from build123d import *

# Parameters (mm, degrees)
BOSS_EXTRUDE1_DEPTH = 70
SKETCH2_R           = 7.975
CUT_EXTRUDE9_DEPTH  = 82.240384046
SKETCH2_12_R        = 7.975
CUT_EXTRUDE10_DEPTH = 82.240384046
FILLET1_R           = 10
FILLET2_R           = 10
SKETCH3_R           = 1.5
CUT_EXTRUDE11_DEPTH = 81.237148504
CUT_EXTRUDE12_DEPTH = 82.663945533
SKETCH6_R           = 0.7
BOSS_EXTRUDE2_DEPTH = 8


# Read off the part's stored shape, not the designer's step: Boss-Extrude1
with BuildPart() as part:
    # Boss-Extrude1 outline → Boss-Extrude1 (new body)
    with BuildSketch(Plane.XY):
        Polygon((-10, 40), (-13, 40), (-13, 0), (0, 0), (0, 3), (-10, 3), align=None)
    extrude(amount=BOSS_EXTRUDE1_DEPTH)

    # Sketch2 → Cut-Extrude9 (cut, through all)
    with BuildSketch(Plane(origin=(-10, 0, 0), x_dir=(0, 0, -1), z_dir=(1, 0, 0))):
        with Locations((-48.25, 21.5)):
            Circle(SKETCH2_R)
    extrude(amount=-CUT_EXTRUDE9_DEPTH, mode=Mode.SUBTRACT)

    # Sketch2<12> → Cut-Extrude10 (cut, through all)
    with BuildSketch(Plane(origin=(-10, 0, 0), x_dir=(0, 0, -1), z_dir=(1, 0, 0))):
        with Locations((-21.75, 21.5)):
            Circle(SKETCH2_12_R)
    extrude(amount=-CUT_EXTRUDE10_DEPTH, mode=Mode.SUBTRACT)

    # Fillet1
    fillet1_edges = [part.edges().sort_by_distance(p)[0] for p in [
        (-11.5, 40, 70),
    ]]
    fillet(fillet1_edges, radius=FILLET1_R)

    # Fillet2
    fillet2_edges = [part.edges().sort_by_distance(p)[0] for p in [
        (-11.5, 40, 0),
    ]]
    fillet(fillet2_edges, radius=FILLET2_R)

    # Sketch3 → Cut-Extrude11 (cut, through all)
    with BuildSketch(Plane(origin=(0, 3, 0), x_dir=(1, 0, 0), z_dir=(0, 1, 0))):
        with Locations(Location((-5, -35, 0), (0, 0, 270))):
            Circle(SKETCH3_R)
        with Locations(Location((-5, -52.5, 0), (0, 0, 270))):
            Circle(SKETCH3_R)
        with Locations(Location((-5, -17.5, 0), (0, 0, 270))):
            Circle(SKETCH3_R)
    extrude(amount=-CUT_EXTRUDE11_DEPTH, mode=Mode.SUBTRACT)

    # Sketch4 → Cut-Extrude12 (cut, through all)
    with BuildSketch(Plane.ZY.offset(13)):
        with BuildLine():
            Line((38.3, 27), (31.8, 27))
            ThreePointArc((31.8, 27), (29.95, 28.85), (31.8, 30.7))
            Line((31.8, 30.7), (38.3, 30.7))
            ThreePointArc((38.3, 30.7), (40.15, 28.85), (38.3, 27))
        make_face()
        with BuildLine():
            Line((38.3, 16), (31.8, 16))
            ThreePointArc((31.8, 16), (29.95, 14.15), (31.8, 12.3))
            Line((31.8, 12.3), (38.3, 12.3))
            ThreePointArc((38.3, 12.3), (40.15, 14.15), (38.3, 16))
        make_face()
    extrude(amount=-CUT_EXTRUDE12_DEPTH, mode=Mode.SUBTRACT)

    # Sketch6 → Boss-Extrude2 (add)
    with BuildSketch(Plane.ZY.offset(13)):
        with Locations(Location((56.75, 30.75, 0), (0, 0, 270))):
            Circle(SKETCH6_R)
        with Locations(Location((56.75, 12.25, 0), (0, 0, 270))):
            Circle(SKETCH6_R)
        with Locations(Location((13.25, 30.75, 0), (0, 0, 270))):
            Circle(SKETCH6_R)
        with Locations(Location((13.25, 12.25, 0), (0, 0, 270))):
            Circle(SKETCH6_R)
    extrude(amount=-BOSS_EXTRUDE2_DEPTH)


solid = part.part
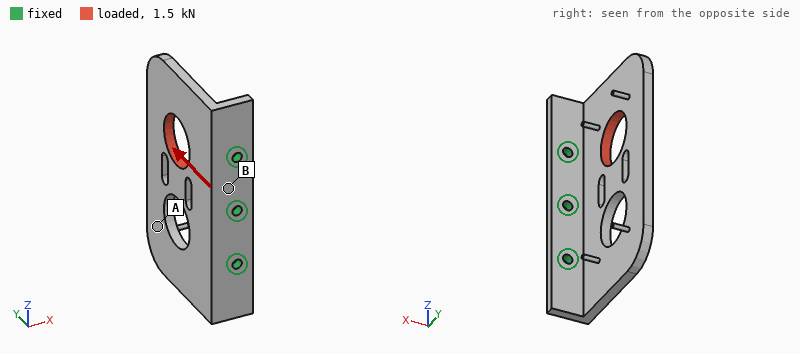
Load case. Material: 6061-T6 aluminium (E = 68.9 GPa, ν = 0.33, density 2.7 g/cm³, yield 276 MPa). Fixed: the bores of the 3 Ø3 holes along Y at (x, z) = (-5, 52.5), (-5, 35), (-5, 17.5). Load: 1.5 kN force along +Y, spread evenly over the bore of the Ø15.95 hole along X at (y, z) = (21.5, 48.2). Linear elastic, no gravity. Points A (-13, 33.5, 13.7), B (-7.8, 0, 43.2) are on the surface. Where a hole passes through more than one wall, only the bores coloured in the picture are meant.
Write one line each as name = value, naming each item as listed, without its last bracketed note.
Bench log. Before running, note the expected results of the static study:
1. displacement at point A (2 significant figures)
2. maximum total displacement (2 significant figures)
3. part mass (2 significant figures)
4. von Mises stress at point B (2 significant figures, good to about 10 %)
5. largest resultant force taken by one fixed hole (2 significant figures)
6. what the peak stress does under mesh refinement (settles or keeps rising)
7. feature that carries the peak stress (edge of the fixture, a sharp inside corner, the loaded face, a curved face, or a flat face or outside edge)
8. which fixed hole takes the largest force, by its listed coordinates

displacement at point A = 0.090 mm
maximum total displacement = 0.23 mm
part mass = 24 g
von Mises stress at point B = 44 MPa
largest resultant force taken by one fixed hole = 1.1 kN
what the peak stress does under mesh refinement = keeps rising
feature that carries the peak stress = edge of the fixture
which fixed hole takes the largest force, by its listed coordinates = (-5, 52.5)
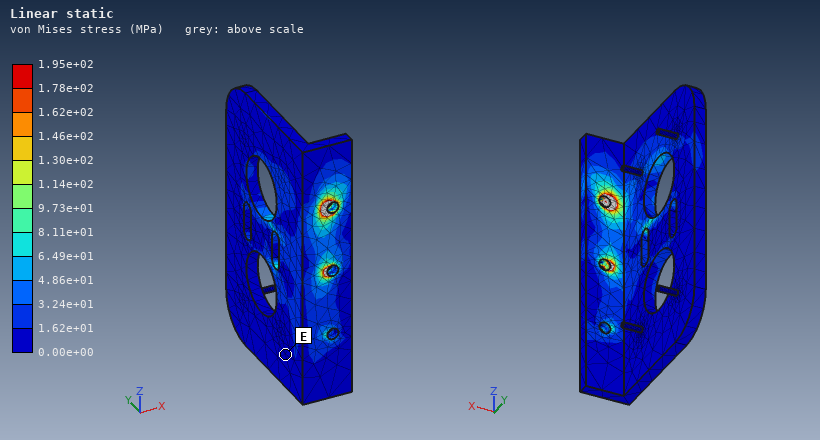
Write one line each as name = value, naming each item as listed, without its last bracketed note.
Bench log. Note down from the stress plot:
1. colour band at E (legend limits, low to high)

colour band at E = 0.00e+00 to 1.62e+01 MPa
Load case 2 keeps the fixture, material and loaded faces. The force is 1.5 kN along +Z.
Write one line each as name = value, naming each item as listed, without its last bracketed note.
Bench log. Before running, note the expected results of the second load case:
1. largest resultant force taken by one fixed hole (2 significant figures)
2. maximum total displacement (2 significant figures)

largest resultant force taken by one fixed hole = 970 N
maximum total displacement = 0.14 mm
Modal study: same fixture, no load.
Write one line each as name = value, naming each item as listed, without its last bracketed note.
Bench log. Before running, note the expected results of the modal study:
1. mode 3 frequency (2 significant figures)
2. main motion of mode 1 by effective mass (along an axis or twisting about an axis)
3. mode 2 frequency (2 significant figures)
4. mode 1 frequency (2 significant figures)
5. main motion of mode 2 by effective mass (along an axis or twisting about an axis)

mode 3 frequency = 4800 Hz
main motion of mode 1 by effective mass = along X
mode 2 frequency = 2100 Hz
mode 1 frequency = 1300 Hz
main motion of mode 2 by effective mass = twisting about Y
